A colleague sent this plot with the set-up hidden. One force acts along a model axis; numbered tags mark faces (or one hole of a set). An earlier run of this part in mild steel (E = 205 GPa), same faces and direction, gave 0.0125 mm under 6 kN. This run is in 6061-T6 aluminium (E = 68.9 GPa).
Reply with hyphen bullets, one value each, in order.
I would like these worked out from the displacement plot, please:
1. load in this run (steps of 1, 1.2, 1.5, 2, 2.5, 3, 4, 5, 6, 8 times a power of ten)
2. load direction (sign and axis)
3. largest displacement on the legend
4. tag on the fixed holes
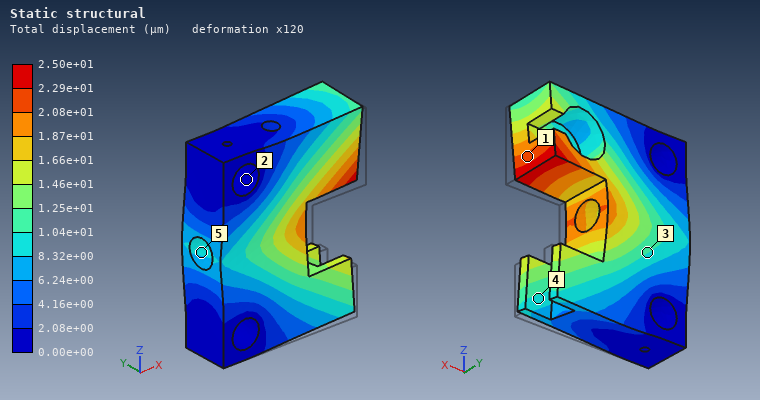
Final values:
- 4 kN
- +Y
- 2.50e+01 µm
- 2
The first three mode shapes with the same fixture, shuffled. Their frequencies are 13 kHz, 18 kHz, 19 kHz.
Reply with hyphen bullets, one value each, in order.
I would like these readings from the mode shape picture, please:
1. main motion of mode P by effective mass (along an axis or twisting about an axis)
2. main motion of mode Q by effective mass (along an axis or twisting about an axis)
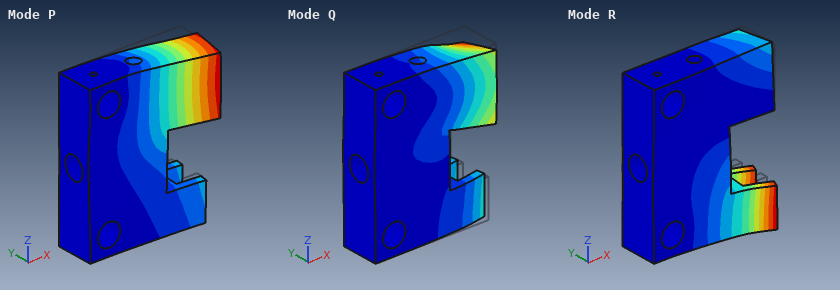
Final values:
- along Y
- along Z
